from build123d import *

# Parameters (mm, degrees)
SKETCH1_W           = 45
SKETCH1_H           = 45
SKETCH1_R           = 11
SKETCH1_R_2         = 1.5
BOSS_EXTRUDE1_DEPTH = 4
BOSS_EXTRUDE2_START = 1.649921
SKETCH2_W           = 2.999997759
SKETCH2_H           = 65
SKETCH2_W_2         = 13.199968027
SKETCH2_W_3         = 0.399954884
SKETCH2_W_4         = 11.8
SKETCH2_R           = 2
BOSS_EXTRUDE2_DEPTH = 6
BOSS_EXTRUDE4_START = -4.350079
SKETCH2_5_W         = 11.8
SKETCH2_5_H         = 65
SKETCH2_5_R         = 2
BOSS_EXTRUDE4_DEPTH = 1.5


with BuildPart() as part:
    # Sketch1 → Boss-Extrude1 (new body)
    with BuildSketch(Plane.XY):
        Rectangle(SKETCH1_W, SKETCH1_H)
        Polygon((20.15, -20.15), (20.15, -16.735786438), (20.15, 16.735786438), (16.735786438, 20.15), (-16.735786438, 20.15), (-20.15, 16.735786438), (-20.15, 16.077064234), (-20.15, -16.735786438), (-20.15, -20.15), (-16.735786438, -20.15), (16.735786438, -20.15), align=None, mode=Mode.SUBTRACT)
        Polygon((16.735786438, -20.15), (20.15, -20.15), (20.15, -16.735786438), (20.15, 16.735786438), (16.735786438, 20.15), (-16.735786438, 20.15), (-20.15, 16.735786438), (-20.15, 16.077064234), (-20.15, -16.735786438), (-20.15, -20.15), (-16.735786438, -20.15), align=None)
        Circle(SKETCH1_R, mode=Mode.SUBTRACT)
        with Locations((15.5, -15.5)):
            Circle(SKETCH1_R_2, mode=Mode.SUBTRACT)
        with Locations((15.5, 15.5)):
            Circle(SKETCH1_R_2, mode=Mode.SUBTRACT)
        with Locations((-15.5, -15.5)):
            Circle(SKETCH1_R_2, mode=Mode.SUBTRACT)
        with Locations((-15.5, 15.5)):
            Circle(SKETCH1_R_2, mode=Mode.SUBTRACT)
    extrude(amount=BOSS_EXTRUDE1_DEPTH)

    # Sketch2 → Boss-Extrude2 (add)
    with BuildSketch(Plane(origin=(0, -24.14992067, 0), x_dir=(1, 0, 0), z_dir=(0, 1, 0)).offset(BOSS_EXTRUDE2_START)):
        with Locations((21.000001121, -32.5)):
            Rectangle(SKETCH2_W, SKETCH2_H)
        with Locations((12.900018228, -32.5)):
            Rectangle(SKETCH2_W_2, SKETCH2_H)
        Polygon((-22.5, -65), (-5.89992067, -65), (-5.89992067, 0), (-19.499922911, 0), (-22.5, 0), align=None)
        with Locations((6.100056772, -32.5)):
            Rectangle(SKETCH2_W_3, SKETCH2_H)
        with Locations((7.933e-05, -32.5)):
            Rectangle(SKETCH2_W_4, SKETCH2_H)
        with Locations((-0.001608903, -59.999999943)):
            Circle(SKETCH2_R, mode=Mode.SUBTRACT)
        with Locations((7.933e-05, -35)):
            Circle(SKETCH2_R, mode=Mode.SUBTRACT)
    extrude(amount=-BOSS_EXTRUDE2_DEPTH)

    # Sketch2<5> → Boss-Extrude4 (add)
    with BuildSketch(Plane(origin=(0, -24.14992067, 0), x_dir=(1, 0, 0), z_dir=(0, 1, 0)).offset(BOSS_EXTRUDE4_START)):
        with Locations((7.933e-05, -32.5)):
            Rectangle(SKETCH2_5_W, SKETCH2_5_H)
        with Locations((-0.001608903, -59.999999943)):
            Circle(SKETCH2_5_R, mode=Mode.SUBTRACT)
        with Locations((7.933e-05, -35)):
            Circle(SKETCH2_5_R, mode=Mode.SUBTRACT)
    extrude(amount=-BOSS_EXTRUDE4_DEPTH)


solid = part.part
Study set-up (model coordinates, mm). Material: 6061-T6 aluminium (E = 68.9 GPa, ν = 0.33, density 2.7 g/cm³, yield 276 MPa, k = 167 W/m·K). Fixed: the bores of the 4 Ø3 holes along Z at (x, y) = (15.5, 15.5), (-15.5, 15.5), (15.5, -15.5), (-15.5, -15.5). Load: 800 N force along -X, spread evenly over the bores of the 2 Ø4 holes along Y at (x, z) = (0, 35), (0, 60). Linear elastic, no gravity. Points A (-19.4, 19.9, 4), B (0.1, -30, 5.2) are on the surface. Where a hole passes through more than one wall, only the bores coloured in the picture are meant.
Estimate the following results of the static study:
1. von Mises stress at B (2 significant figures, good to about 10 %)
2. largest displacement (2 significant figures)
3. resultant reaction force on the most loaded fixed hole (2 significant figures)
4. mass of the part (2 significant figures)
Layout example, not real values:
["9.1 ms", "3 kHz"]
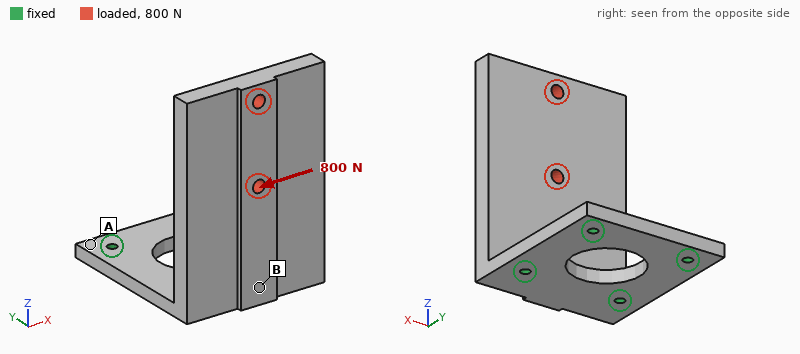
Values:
["26 MPa", "0.15 mm", "1.2 kN", "67 g"]
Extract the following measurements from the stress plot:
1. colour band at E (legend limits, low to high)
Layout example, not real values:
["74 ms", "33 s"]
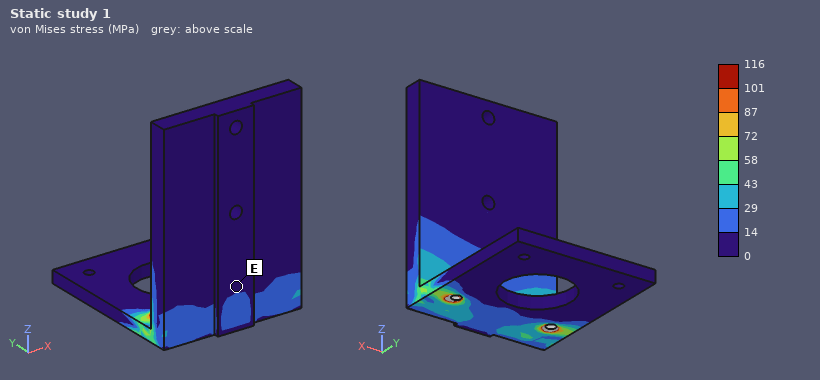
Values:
["0 to 14 MPa"]
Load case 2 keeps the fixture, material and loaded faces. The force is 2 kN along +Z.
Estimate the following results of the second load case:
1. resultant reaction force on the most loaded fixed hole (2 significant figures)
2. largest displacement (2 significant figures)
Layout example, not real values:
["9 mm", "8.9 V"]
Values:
["1.1 kN", "0.57 mm"]
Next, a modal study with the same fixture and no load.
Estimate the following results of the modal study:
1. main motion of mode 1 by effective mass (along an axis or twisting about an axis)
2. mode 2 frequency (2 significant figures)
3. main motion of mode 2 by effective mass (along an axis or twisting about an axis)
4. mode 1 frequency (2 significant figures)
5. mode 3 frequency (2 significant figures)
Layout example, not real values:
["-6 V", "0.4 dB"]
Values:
["along Y", "2400 Hz", "along X", "700 Hz", "3900 Hz"]
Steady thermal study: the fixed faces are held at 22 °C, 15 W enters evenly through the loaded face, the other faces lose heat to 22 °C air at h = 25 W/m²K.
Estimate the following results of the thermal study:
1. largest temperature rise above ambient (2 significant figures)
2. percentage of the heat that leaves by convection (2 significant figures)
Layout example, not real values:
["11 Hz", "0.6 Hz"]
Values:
["20 K", "15 %"]
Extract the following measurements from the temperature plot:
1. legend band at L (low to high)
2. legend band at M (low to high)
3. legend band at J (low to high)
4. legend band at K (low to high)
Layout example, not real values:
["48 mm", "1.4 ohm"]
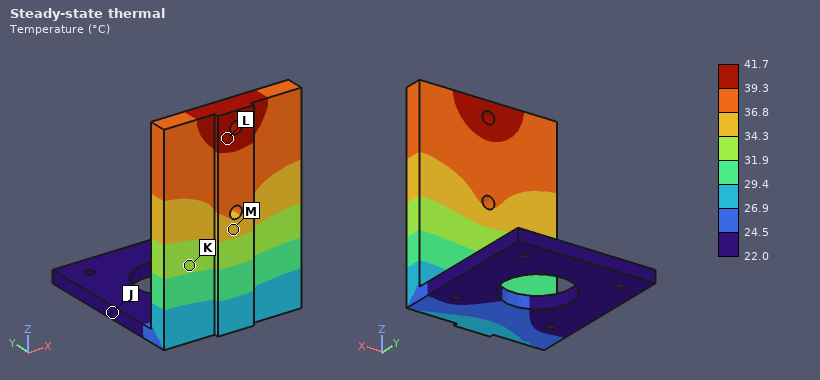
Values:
["39.3 to 41.7 °C", "34.3 to 36.8 °C", "22.0 to 24.5 °C", "31.9 to 34.3 °C"]
